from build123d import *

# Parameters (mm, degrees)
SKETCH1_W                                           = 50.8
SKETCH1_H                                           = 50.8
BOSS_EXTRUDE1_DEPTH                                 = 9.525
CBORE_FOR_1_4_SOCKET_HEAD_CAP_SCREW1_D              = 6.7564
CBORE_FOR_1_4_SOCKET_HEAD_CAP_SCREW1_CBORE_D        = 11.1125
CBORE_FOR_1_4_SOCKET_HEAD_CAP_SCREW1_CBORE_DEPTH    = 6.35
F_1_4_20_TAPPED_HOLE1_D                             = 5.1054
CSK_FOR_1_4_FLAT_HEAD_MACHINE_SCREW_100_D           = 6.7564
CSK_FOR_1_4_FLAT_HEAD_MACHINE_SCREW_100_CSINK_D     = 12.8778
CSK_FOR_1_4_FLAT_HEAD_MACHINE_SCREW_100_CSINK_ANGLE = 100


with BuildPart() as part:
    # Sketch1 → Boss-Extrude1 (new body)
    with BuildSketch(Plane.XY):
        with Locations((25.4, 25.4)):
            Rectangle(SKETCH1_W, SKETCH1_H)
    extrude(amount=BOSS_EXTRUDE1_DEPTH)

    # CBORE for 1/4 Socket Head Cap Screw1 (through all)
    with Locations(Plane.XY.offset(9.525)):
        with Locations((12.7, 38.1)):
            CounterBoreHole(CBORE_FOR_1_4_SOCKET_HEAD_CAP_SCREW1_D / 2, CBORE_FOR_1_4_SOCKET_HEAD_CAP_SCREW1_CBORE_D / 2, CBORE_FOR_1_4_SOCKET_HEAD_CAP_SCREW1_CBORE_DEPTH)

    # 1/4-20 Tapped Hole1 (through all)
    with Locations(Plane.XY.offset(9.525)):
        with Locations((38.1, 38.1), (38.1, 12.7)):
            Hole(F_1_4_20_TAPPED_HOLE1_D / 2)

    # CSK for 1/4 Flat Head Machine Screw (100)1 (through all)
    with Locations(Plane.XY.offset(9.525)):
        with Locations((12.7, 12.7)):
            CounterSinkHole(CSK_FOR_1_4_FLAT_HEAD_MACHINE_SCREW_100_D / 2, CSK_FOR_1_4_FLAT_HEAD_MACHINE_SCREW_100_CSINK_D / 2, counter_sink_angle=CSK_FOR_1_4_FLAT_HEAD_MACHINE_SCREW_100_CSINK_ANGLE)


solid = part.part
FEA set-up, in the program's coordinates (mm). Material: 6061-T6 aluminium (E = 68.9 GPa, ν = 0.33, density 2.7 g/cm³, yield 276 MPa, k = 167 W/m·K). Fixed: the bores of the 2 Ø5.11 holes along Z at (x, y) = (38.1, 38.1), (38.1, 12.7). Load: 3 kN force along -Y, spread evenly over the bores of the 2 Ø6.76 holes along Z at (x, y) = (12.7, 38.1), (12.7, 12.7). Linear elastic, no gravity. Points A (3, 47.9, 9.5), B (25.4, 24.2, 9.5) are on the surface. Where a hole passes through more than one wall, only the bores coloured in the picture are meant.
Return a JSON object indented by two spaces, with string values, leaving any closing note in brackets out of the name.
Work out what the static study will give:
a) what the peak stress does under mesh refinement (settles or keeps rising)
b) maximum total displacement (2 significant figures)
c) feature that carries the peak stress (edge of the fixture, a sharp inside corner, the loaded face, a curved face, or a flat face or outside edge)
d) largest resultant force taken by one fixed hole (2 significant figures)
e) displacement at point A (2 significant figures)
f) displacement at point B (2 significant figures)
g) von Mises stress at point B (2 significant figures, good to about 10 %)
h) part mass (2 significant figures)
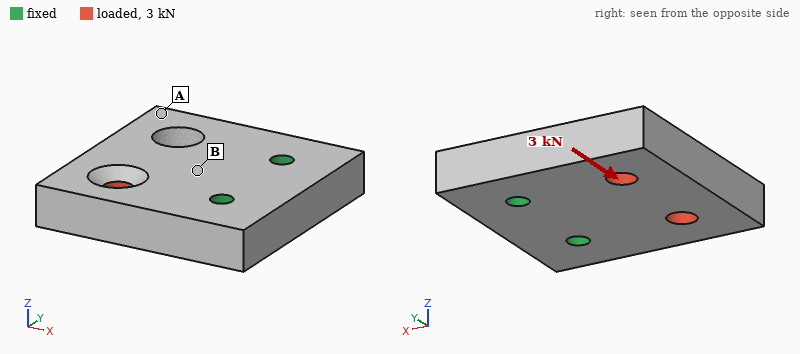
{
  "what the peak stress does under mesh refinement": "keeps rising",
  "maximum total displacement": "21 µm",
  "feature that carries the peak stress": "edge of the fixture",
  "largest resultant force taken by one fixed hole": "3.0 kN",
  "displacement at point A": "17 µm",
  "displacement at point B": "5.0 µm",
  "von Mises stress at point B": "14 MPa",
  "part mass": "62 g"
}
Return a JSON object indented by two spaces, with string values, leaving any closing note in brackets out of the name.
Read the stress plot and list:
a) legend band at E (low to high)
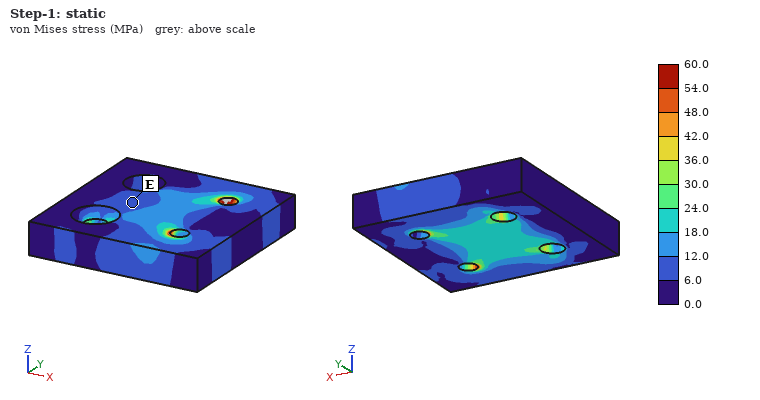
{
  "legend band at E": "6.0 to 12.0 MPa"
}
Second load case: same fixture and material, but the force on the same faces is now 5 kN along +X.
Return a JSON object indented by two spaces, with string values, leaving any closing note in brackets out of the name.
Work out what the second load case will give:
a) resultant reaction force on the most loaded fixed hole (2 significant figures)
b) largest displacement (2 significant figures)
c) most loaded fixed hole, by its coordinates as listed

{
  "resultant reaction force on the most loaded fixed hole": "3.4 kN",
  "largest displacement": "28 µm",
  "most loaded fixed hole, by its coordinates as listed": "(38.1, 12.7)"
}
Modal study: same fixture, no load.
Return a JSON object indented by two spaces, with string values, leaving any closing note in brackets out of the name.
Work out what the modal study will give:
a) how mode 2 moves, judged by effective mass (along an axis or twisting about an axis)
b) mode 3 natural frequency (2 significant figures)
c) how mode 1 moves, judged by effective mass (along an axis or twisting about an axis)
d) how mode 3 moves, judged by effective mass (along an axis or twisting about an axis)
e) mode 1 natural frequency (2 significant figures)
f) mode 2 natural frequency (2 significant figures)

{
  "how mode 2 moves, judged by effective mass": "twisting about X",
  "mode 3 natural frequency": "13 kHz",
  "how mode 1 moves, judged by effective mass": "along Z",
  "how mode 3 moves, judged by effective mass": "along Y",
  "mode 1 natural frequency": "5000 Hz",
  "mode 2 natural frequency": "8700 Hz"
}
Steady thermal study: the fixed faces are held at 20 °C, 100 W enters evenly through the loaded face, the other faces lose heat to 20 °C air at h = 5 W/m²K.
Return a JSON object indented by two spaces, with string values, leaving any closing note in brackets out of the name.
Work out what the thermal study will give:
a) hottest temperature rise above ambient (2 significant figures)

{
  "hottest temperature rise above ambient": "48 K"
}
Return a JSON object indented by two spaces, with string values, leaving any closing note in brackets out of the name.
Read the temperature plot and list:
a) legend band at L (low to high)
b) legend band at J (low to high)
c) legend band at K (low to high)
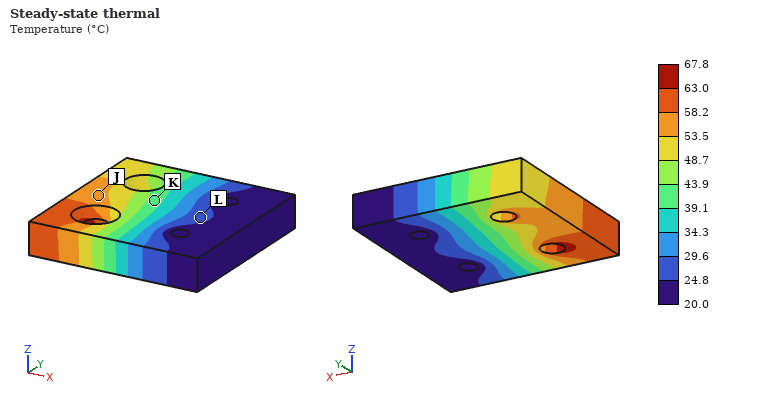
{
  "legend band at L": "24.8 to 29.6 °C",
  "legend band at J": "53.5 to 58.2 °C",
  "legend band at K": "39.1 to 43.9 °C"
}
